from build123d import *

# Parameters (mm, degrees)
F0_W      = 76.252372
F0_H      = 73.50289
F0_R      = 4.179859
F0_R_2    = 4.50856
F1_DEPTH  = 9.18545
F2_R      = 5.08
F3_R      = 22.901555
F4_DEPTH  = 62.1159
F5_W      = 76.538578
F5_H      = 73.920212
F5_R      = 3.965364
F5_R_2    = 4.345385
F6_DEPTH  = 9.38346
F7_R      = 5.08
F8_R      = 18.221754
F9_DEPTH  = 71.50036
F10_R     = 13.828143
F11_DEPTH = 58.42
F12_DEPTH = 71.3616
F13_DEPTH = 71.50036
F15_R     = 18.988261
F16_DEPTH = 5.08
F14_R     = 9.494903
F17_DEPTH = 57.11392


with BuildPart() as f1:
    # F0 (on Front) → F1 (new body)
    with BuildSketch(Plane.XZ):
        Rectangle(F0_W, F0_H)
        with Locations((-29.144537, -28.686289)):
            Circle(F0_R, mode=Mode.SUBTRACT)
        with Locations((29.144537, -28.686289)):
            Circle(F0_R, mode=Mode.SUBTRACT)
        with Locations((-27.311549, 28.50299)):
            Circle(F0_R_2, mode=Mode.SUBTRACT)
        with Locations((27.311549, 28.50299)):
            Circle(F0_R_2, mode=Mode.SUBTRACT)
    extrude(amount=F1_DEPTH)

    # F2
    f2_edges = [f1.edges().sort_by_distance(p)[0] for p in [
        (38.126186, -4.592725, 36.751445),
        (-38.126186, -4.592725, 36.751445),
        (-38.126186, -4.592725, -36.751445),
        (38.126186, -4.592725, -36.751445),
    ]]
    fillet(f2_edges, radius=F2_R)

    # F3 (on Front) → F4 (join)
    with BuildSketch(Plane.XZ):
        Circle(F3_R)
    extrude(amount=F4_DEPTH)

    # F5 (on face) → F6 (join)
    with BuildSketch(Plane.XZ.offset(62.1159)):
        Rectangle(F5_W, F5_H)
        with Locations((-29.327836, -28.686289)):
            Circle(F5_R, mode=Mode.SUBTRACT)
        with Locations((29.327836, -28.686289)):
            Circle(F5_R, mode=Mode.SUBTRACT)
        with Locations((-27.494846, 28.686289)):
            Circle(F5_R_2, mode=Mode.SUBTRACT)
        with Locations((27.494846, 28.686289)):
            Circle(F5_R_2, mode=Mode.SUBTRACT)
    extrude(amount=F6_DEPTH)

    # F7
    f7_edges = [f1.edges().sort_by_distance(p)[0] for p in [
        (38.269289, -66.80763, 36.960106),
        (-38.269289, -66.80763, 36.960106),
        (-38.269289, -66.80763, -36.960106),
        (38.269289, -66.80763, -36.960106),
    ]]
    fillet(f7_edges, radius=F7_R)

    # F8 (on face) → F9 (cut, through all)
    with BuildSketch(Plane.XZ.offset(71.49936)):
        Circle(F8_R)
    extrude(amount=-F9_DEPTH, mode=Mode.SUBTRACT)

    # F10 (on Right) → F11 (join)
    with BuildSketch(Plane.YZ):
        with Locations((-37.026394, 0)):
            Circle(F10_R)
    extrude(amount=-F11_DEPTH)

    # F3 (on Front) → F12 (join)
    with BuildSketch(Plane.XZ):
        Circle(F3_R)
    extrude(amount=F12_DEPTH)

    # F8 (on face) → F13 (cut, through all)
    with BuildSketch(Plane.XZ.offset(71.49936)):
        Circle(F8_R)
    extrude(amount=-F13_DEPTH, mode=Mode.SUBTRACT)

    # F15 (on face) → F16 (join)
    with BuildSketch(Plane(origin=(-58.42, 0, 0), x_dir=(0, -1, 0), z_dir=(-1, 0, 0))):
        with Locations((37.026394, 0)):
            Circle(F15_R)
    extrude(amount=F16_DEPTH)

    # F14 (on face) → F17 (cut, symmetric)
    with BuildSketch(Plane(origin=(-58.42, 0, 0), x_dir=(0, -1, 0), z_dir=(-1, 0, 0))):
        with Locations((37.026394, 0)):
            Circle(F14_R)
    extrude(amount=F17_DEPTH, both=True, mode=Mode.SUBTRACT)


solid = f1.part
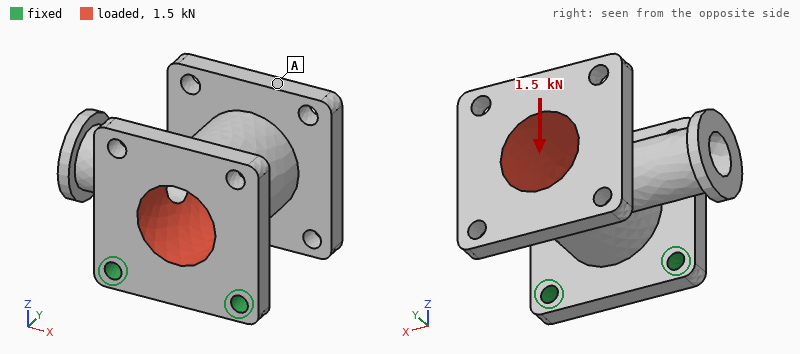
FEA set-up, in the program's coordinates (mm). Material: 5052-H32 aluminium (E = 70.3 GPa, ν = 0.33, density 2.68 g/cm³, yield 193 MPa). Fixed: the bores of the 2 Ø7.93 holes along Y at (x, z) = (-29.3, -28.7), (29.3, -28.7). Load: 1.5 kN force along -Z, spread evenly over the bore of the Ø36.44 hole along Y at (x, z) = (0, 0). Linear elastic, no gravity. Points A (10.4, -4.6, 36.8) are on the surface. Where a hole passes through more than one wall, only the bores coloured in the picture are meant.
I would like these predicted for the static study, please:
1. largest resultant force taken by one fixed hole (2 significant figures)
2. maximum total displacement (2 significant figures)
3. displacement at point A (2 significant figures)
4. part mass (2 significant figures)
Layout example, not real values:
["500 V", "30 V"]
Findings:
["830 N", "0.28 mm", "0.27 mm", "340 g"]
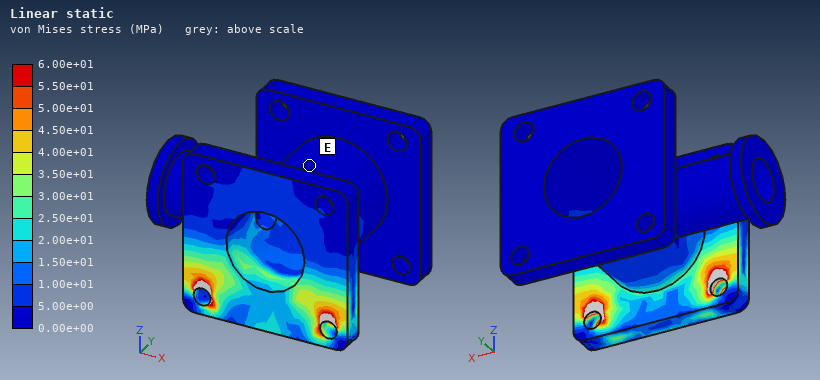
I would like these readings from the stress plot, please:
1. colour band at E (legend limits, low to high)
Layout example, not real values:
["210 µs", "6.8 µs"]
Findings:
["0.00e+00 to 5.00e+00 MPa"]
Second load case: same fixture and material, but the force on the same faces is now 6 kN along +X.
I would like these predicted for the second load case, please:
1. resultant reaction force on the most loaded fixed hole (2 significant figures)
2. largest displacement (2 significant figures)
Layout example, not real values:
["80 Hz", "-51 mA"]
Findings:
["5.3 kN", "0.25 mm"]
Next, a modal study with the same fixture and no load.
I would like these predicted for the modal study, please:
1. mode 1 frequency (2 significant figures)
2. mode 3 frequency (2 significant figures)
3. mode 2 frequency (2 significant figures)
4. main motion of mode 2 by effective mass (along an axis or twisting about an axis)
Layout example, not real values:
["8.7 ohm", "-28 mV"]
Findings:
["670 Hz", "3100 Hz", "1400 Hz", "along X"]
